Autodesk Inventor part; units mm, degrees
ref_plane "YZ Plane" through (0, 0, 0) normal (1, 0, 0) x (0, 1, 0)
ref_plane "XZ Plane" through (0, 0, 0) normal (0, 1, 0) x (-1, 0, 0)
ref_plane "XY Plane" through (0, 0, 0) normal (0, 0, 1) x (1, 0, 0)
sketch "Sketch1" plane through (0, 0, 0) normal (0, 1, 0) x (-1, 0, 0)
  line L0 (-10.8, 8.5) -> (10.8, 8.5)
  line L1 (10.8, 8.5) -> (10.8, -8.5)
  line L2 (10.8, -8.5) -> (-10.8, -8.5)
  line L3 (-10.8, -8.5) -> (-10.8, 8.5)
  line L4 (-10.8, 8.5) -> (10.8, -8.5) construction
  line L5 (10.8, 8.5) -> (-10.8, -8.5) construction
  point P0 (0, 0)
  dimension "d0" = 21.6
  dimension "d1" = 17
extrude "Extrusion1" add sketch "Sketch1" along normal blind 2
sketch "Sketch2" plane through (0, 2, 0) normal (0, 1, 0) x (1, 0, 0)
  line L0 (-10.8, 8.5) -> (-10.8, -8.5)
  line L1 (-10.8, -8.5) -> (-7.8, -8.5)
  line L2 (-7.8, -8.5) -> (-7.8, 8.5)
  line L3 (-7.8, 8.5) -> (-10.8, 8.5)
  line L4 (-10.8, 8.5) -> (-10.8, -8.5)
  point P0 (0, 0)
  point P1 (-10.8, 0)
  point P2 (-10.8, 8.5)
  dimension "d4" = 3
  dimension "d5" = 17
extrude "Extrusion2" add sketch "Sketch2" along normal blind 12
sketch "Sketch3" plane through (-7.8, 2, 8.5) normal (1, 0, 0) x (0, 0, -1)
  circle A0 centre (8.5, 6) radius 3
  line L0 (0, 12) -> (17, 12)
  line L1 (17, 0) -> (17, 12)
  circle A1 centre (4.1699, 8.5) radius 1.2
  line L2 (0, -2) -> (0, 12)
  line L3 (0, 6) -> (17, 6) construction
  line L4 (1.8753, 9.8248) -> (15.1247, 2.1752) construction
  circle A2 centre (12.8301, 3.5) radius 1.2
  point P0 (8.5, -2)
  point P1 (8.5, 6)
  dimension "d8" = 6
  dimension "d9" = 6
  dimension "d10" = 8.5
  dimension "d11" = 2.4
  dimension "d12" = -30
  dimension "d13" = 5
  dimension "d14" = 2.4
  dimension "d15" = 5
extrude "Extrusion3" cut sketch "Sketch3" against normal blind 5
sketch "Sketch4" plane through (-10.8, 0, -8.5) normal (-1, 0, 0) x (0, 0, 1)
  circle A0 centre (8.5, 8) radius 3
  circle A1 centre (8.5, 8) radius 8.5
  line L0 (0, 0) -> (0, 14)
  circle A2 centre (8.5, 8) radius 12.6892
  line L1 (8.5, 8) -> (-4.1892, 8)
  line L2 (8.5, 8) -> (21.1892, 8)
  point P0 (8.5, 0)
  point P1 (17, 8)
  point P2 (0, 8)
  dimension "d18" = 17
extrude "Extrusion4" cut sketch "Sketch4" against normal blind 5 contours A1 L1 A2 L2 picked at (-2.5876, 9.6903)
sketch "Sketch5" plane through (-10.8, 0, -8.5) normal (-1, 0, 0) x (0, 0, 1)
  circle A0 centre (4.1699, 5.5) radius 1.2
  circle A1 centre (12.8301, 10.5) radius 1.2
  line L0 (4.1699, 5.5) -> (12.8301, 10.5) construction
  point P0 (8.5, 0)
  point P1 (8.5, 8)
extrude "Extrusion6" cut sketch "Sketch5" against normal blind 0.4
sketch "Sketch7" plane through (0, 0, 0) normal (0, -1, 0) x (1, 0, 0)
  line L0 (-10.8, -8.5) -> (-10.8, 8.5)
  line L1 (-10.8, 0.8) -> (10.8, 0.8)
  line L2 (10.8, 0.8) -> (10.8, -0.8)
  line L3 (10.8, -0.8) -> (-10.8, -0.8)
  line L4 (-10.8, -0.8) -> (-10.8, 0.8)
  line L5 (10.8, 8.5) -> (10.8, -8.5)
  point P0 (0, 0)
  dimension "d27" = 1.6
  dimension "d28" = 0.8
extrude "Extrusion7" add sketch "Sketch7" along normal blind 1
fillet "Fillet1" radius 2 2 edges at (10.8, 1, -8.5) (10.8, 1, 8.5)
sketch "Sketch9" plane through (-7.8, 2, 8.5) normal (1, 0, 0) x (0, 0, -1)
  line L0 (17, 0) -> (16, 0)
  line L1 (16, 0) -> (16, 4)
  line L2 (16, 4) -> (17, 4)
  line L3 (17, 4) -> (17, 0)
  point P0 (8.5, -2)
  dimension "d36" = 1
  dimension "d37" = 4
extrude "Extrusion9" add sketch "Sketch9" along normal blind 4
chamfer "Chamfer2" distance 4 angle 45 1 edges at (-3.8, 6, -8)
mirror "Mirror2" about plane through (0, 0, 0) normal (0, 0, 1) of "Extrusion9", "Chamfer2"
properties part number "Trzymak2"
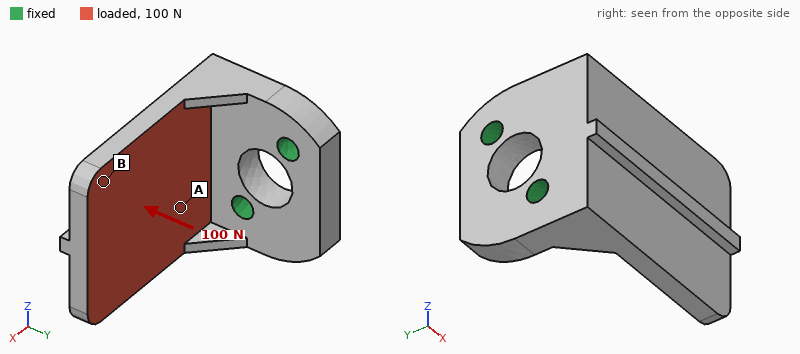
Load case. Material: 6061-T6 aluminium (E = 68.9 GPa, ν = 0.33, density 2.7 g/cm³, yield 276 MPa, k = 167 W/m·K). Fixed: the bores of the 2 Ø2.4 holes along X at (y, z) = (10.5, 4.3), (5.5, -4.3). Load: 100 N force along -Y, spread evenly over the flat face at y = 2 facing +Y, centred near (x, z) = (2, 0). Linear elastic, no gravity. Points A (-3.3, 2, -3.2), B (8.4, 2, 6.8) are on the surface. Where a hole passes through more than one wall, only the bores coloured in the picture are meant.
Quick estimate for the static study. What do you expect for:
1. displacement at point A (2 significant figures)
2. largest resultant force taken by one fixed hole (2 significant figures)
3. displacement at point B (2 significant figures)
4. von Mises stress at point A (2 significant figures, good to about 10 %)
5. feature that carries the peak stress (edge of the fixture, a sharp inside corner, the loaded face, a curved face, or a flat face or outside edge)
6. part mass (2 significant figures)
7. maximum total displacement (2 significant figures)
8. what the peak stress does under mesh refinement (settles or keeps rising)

0.021 mm
64 N
0.10 mm
34 MPa
a sharp inside corner
3.4 g
0.12 mm
keeps rising
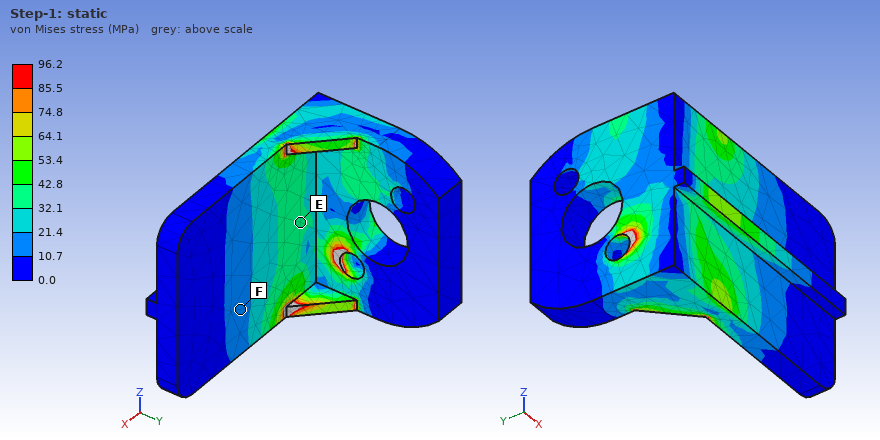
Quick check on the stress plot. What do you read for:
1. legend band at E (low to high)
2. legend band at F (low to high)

32.1 to 42.8 MPa
10.7 to 21.4 MPa
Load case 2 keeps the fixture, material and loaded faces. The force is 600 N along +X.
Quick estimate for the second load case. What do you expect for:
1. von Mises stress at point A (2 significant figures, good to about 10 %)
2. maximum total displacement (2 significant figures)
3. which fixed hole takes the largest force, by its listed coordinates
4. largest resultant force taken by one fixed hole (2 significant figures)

45 MPa
57 µm
(5.5, -4.3)
440 N
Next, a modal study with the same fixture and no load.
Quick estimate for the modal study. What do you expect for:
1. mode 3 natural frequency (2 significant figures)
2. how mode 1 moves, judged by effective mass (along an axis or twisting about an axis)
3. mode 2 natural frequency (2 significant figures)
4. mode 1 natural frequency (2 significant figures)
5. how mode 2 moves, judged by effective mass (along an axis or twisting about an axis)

13 kHz
along Y
8300 Hz
4300 Hz
along Z
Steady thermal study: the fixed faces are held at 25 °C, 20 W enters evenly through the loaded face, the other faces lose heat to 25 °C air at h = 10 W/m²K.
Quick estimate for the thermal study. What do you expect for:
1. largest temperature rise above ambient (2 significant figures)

47 K
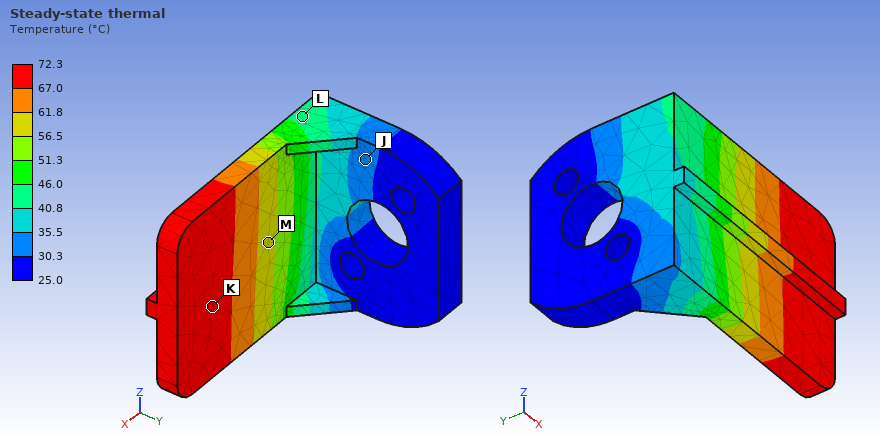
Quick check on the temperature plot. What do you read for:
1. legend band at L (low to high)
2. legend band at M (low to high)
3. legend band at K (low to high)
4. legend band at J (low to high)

40.8 to 46.0 °C
56.5 to 61.8 °C
67.0 to 72.3 °C
30.3 to 35.5 °C
